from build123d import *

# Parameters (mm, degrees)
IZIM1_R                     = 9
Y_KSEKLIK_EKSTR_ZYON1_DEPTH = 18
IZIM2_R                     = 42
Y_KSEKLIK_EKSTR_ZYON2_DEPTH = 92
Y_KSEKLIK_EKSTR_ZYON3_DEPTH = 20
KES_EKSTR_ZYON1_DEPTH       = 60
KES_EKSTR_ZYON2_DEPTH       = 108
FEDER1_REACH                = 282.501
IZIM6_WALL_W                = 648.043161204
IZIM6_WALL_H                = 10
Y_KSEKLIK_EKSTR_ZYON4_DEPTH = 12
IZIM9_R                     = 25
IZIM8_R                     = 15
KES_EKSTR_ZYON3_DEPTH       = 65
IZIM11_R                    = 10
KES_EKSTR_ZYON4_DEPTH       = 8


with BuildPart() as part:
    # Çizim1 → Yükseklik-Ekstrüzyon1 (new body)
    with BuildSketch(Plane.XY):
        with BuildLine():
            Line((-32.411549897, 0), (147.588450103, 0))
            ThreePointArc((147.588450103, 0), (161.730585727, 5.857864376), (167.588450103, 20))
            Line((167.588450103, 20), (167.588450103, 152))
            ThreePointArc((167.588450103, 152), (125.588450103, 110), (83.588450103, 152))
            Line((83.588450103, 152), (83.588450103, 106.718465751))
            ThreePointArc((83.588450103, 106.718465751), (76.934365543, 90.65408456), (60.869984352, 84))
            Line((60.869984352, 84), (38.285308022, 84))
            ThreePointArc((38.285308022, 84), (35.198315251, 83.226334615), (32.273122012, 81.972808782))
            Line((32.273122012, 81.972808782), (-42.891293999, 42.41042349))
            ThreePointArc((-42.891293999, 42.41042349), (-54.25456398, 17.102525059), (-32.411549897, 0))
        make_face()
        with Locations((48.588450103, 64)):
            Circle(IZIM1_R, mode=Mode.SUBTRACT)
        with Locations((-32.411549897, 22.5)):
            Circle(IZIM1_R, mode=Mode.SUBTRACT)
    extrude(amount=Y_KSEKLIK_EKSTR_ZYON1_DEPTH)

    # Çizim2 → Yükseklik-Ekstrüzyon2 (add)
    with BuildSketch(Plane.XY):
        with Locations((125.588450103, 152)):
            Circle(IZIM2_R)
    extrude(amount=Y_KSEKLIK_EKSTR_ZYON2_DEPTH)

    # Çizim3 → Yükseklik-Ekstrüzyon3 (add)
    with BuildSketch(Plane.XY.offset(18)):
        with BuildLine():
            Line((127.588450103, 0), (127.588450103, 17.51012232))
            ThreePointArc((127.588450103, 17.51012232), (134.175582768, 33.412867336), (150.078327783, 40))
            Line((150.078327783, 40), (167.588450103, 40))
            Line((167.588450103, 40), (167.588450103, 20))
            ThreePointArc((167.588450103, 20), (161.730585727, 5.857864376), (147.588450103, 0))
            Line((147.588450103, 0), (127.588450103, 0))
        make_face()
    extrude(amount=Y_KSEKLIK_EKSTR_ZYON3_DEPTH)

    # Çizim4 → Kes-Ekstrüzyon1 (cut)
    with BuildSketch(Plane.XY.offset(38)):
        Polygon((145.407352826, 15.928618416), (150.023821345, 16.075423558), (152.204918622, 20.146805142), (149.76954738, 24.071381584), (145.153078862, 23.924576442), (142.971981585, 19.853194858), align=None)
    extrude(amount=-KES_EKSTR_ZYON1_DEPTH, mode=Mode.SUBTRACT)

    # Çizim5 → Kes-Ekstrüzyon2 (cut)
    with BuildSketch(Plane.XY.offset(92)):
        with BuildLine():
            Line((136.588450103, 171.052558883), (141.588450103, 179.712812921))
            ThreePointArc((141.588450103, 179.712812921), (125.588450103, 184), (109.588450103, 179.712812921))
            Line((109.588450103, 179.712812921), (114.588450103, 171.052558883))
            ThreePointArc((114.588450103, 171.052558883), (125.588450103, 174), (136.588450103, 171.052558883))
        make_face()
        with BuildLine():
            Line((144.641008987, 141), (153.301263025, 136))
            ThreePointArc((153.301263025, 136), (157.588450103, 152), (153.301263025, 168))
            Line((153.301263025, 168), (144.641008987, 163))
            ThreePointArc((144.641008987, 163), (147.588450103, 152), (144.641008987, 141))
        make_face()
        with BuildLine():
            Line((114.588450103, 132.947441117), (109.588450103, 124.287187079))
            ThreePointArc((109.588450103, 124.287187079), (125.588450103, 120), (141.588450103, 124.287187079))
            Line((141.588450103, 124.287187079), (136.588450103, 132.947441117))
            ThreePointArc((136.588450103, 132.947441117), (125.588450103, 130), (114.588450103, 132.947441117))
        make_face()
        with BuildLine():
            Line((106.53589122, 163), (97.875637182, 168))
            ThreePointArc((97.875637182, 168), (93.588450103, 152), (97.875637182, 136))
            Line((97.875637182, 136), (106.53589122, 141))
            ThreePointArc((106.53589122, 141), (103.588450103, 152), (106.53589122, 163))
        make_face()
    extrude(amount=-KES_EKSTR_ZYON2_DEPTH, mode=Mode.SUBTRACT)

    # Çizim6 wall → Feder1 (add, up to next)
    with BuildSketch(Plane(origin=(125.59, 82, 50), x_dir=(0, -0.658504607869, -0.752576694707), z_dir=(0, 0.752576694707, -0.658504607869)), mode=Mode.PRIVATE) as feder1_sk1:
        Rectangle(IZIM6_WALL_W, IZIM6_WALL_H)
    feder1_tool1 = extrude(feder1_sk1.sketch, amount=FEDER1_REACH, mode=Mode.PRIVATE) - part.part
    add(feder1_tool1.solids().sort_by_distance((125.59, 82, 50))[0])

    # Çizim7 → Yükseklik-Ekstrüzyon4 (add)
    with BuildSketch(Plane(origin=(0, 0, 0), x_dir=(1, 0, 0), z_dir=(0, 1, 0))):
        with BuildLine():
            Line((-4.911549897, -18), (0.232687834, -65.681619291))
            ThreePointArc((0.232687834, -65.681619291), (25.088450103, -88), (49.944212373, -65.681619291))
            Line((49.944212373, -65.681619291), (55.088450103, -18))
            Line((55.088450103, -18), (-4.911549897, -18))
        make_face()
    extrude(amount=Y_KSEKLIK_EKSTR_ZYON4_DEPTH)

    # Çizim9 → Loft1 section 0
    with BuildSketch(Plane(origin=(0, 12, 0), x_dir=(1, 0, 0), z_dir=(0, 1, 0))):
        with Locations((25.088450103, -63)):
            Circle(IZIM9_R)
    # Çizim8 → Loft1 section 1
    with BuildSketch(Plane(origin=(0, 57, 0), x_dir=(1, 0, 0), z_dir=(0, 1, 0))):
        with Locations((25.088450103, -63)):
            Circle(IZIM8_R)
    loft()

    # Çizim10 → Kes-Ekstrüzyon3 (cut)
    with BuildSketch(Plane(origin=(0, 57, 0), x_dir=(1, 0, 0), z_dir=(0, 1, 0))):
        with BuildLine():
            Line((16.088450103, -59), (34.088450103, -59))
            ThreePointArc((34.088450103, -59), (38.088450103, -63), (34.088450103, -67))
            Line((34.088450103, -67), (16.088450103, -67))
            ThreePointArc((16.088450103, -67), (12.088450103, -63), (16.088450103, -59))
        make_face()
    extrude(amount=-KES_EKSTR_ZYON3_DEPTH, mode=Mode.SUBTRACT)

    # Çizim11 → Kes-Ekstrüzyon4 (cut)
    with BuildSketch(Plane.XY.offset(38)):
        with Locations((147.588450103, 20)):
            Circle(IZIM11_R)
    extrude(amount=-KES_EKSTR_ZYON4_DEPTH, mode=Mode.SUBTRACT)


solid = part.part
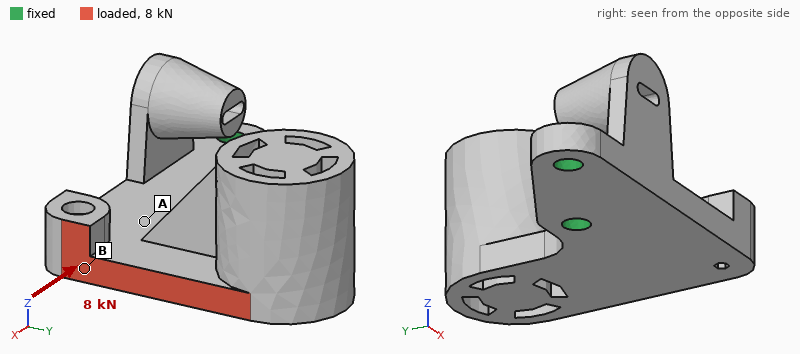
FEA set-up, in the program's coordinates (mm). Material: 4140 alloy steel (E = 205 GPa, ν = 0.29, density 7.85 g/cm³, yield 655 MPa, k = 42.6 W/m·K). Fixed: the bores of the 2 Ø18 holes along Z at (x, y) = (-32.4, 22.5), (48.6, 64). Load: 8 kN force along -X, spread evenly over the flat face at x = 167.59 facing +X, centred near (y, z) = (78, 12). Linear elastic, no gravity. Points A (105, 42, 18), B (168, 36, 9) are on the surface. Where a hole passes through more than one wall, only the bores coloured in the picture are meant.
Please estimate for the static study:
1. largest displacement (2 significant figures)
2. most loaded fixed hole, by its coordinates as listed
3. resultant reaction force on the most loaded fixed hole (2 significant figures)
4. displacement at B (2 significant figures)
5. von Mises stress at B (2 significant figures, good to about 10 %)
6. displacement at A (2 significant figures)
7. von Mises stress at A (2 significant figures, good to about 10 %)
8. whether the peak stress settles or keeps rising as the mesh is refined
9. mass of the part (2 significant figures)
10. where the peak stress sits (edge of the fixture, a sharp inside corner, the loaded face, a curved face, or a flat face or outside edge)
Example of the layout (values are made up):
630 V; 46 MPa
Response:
32 µm; (48.6, 64); 8.8 kN; 19 µm; 3.5 MPa; 5.9 µm; 8.6 MPa; keeps rising; 6.9 kg; edge of the fixture
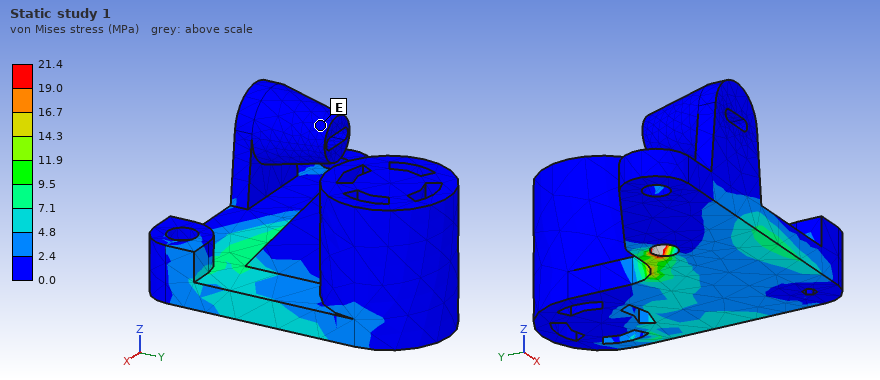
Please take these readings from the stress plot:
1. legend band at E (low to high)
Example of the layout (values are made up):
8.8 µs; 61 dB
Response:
0.0 to 2.4 MPa
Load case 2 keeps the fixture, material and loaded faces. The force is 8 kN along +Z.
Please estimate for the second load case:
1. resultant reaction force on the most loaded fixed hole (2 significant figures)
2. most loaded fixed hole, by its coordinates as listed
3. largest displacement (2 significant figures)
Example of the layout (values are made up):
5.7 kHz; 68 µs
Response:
12 kN; (48.6, 64); 0.75 mm
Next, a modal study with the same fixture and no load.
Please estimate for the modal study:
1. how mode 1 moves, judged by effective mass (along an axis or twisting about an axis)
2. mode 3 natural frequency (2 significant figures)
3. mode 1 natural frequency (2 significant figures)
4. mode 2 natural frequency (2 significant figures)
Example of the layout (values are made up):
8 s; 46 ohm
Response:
along Z; 1000 Hz; 290 Hz; 490 Hz
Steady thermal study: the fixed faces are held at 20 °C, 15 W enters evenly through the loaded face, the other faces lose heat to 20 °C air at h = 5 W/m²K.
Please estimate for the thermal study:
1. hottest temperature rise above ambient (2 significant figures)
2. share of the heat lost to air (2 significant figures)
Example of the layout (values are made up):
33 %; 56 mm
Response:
16 K; 35 %
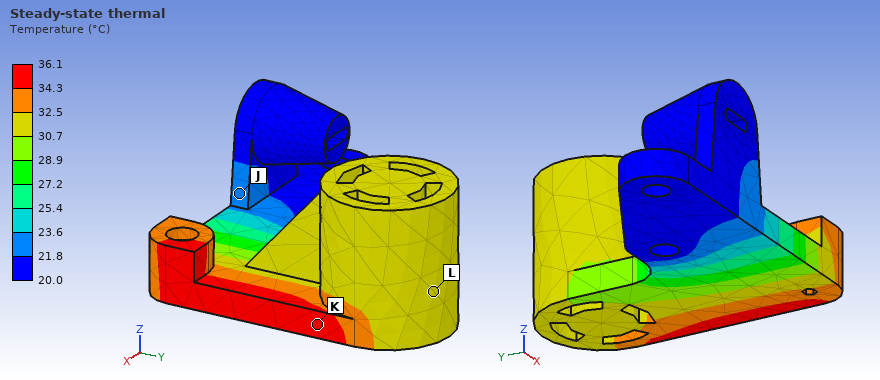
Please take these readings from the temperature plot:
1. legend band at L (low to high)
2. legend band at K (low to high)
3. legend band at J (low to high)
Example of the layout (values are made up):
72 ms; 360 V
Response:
30.7 to 32.5 °C; 34.3 to 36.1 °C; 21.8 to 23.6 °C
